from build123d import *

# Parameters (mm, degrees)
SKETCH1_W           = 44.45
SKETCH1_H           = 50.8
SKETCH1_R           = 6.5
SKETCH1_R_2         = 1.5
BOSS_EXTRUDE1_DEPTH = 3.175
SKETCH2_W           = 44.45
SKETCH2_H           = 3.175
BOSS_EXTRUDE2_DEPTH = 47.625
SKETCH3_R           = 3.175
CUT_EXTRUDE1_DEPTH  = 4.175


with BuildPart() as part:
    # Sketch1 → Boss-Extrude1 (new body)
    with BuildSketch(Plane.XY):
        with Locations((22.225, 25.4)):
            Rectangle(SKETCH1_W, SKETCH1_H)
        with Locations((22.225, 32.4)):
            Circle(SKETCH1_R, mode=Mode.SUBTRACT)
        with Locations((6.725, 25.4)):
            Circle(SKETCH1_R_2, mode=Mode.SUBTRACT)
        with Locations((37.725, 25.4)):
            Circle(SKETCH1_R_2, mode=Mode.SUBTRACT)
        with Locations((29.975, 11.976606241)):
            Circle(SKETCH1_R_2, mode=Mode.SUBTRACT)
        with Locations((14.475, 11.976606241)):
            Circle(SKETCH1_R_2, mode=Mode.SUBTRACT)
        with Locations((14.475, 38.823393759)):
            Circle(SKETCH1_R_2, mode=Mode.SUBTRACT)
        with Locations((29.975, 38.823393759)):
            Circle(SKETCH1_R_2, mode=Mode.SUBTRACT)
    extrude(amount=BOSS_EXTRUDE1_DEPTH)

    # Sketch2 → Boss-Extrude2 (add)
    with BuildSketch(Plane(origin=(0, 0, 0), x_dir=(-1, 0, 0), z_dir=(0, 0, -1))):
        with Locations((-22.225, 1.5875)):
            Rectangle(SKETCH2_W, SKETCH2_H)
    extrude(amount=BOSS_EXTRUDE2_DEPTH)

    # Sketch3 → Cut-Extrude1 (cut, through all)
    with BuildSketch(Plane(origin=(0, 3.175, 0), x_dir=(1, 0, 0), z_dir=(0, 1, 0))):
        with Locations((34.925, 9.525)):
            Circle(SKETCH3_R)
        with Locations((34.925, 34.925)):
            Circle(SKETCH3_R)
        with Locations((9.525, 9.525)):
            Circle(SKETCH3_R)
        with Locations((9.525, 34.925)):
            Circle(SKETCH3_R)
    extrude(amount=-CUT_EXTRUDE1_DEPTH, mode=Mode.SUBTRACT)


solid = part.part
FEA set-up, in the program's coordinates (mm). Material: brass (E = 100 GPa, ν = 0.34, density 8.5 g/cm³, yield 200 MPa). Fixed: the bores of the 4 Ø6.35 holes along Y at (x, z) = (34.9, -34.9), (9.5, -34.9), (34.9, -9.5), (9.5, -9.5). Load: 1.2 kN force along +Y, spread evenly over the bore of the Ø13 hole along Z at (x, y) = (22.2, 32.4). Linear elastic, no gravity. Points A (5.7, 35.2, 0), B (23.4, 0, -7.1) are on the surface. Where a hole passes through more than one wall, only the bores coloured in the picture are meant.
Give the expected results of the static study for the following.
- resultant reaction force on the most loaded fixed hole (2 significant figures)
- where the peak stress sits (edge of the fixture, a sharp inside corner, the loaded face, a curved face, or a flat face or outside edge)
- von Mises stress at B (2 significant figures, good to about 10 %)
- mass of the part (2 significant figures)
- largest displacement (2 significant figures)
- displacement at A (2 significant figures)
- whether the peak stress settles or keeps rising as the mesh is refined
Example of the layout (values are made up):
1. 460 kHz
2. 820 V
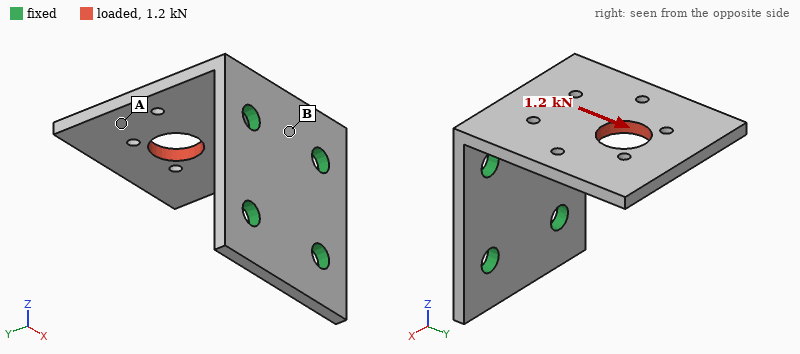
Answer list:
1. 620 N
2. edge of the fixture
3. 50 MPa
4. 110 g
5. 0.22 mm
6. 0.15 mm
7. keeps rising
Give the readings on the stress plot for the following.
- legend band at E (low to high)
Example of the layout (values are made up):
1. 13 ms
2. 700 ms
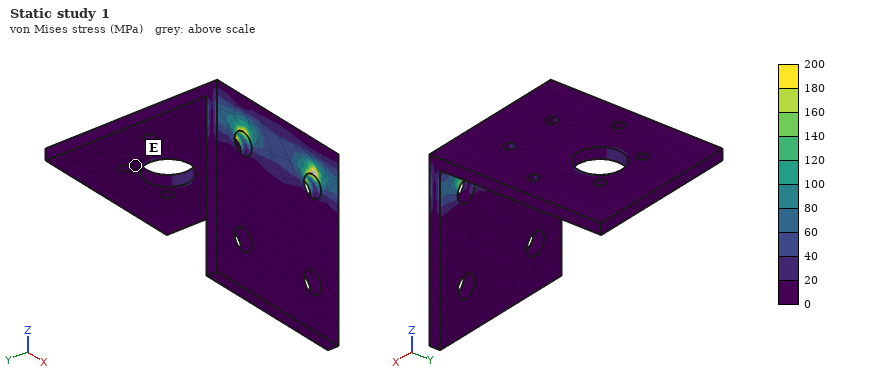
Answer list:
1. 0 to 20 MPa
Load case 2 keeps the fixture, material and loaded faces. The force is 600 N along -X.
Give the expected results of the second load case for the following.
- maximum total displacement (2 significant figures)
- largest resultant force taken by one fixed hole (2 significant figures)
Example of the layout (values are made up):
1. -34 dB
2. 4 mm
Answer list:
1. 0.11 mm
2. 740 N
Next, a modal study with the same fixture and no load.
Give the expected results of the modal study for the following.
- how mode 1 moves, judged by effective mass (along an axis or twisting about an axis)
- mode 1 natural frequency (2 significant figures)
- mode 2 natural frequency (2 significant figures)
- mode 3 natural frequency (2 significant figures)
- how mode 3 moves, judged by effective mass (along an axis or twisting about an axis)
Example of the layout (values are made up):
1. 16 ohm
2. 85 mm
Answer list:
1. along Z
2. 590 Hz
3. 1600 Hz
4. 2400 Hz
5. along X
